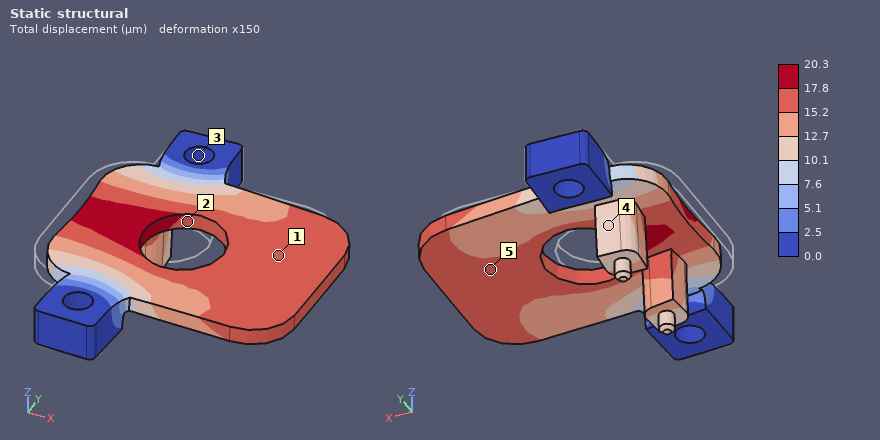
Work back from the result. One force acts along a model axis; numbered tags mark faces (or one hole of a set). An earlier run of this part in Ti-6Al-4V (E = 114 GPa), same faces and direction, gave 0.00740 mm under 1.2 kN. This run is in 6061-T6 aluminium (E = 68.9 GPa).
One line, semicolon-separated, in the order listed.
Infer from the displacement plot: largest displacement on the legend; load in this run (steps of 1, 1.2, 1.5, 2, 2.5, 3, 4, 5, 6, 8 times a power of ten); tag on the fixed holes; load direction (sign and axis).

20.3 µm; 2 kN; 3; +X
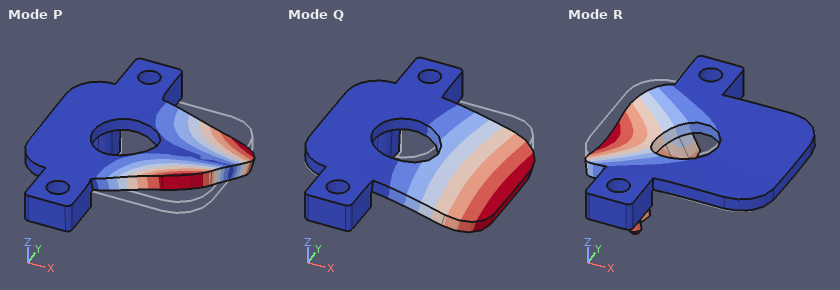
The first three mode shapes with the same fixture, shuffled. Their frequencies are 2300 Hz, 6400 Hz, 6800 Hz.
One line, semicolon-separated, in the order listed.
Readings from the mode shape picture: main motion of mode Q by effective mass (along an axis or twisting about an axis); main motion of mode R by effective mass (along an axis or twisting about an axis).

along Z; along Z
